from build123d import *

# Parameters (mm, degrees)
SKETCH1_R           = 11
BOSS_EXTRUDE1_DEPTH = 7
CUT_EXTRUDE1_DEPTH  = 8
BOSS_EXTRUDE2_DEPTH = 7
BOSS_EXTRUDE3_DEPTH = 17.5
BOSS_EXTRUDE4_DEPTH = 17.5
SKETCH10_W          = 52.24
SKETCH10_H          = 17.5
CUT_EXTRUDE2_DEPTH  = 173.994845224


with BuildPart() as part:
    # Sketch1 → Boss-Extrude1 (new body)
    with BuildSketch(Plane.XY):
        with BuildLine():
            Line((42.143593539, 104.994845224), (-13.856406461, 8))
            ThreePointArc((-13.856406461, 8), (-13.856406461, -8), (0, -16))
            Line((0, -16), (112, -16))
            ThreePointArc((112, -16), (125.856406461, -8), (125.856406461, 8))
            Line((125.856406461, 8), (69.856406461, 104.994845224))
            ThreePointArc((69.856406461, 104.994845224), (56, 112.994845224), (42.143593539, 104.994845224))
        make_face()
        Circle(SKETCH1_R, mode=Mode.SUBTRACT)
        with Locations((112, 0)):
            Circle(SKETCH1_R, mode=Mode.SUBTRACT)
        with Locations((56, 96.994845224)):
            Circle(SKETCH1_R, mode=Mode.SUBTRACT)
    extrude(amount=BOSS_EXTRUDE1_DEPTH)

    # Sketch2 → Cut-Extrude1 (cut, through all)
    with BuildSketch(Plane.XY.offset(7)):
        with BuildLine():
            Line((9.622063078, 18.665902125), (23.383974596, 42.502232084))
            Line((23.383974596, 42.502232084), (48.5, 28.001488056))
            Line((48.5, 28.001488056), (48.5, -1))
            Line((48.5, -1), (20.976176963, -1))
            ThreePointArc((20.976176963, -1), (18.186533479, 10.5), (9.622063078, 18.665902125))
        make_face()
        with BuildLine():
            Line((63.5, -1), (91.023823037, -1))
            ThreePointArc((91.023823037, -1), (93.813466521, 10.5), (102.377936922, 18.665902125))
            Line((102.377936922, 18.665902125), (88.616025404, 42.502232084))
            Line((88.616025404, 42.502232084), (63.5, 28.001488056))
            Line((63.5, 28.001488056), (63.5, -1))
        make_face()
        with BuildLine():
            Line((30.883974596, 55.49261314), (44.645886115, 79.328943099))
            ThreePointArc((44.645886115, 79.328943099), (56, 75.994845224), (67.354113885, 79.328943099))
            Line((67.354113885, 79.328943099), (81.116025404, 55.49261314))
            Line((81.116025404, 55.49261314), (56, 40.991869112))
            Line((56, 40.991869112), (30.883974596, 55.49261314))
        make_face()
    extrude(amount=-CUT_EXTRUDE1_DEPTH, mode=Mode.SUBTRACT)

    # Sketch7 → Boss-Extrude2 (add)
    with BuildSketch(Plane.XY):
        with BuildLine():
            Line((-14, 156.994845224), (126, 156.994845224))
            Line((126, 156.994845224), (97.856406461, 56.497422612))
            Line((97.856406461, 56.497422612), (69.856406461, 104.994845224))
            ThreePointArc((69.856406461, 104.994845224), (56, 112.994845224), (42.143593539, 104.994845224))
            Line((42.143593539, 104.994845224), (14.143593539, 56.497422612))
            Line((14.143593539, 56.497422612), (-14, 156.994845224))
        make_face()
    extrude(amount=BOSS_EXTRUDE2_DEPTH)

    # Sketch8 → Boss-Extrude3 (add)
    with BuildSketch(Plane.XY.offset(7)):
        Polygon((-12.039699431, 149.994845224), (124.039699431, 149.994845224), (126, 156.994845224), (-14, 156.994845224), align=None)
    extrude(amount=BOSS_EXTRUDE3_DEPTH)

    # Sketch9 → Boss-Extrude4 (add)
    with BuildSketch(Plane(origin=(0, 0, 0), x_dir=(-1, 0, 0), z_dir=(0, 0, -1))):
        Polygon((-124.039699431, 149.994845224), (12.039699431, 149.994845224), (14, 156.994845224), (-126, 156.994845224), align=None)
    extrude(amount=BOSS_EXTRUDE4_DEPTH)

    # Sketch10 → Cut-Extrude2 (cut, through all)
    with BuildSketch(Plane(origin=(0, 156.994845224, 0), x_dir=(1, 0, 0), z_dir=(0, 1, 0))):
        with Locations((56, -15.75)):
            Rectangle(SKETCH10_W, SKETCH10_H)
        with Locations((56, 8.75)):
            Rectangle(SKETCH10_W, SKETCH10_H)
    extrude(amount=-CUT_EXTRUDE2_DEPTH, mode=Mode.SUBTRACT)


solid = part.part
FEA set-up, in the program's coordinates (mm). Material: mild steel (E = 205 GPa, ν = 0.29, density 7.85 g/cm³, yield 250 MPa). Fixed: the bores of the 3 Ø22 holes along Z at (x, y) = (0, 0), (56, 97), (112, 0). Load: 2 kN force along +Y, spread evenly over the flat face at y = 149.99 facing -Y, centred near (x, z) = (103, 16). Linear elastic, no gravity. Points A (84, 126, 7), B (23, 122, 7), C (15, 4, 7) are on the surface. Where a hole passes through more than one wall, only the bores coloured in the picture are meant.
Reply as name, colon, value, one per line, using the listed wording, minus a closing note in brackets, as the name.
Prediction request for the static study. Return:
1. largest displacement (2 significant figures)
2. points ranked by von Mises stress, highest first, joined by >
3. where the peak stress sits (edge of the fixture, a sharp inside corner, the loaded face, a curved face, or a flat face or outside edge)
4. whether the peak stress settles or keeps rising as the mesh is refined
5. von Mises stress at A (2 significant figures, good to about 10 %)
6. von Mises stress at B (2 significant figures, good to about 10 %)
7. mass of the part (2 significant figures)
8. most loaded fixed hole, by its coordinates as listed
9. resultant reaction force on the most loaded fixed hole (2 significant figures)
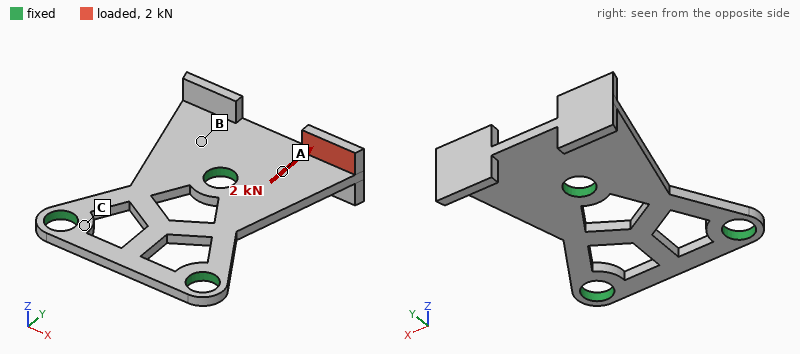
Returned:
largest displacement: 0.15 mm
points ranked by von Mises stress, highest first, joined by >: A > B > C
where the peak stress sits: a sharp inside corner
whether the peak stress settles or keeps rising as the mesh is refined: keeps rising
von Mises stress at A: 41 MPa
von Mises stress at B: 12 MPa
mass of the part: 1.0 kg
most loaded fixed hole, by its coordinates as listed: (56, 97)
resultant reaction force on the most loaded fixed hole: 1.7 kN
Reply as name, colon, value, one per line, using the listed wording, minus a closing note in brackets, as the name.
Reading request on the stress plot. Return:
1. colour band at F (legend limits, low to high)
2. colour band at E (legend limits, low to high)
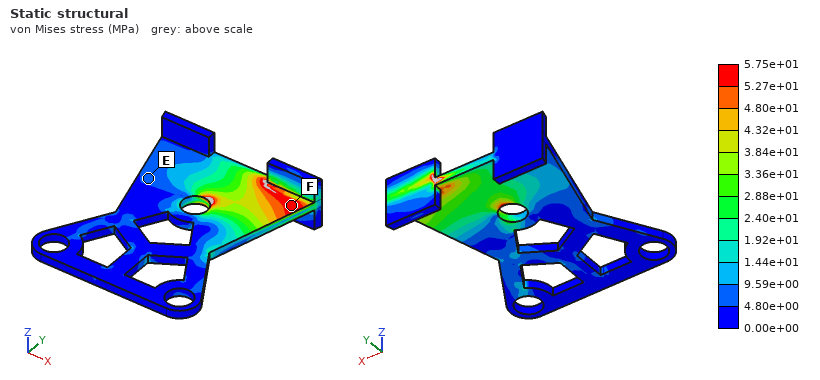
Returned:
colour band at F: 5.27e+01 to 5.75e+01 MPa
colour band at E: 4.80e+00 to 9.59e+00 MPa
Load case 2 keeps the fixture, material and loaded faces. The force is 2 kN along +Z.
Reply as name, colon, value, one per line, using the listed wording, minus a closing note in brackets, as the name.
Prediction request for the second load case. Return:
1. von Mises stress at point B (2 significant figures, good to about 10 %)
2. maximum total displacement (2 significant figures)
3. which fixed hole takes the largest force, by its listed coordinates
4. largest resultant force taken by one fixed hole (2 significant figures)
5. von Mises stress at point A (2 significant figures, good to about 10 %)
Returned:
von Mises stress at point B: 38 MPa
maximum total displacement: 0.59 mm
which fixed hole takes the largest force, by its listed coordinates: (56, 97)
largest resultant force taken by one fixed hole: 2.2 kN
von Mises stress at point A: 87 MPa
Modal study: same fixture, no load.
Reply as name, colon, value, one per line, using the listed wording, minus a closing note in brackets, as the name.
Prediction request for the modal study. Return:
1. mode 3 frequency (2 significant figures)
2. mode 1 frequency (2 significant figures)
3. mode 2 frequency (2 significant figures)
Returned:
mode 3 frequency: 2200 Hz
mode 1 frequency: 870 Hz
mode 2 frequency: 890 Hz
